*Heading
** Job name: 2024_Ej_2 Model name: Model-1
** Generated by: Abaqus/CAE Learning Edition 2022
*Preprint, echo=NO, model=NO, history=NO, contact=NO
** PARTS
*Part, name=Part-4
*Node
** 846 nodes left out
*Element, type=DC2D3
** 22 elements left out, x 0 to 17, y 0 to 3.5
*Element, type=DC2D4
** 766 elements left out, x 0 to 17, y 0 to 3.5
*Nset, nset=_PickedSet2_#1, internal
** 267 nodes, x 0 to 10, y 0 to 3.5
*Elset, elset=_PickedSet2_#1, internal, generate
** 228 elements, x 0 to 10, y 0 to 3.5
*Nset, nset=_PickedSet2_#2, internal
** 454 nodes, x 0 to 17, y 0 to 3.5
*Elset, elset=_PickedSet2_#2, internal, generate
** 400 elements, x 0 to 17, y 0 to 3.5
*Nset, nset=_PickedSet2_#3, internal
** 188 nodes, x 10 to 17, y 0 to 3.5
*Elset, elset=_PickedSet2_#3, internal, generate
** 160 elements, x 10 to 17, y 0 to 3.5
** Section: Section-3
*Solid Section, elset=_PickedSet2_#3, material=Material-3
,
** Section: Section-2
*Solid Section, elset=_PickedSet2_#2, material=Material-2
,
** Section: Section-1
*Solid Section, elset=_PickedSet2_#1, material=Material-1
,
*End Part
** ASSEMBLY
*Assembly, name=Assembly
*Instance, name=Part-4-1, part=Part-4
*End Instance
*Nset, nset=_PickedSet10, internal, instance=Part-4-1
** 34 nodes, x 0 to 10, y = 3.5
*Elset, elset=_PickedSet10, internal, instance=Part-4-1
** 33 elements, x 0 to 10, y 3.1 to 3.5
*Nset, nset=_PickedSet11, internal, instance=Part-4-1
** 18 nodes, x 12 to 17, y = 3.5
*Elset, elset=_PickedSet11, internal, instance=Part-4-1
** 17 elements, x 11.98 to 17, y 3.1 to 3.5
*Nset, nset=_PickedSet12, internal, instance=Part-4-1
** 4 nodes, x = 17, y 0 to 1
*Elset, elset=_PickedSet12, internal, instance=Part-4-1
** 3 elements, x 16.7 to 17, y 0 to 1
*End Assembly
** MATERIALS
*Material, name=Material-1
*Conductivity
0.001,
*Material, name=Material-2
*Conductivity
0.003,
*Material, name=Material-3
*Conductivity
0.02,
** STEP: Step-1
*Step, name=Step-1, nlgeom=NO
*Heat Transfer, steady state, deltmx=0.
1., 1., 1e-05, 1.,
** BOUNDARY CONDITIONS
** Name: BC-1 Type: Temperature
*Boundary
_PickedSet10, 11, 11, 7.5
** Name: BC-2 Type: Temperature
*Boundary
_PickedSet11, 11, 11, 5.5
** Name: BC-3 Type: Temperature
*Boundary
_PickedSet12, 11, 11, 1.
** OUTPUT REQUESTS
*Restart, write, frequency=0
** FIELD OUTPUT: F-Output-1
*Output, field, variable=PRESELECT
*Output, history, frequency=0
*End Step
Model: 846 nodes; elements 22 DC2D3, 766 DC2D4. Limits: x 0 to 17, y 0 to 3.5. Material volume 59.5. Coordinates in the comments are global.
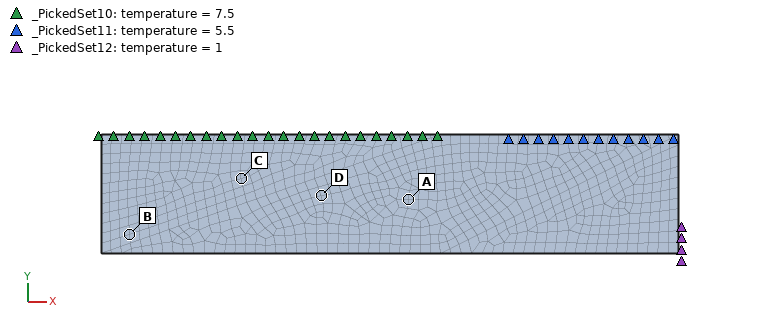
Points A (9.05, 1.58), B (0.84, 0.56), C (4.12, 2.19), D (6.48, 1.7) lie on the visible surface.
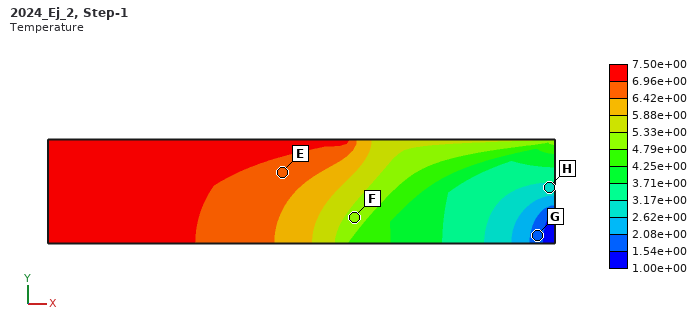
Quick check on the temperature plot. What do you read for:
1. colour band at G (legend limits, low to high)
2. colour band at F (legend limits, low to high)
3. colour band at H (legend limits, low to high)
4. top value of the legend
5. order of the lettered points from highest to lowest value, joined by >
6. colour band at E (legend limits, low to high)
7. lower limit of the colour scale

1.54e+00 to 2.08e+00
4.79e+00 to 5.33e+00
2.62e+00 to 3.17e+00
7.50e+00
E > F > H > G
6.42e+00 to 6.96e+00
1.00e+00
